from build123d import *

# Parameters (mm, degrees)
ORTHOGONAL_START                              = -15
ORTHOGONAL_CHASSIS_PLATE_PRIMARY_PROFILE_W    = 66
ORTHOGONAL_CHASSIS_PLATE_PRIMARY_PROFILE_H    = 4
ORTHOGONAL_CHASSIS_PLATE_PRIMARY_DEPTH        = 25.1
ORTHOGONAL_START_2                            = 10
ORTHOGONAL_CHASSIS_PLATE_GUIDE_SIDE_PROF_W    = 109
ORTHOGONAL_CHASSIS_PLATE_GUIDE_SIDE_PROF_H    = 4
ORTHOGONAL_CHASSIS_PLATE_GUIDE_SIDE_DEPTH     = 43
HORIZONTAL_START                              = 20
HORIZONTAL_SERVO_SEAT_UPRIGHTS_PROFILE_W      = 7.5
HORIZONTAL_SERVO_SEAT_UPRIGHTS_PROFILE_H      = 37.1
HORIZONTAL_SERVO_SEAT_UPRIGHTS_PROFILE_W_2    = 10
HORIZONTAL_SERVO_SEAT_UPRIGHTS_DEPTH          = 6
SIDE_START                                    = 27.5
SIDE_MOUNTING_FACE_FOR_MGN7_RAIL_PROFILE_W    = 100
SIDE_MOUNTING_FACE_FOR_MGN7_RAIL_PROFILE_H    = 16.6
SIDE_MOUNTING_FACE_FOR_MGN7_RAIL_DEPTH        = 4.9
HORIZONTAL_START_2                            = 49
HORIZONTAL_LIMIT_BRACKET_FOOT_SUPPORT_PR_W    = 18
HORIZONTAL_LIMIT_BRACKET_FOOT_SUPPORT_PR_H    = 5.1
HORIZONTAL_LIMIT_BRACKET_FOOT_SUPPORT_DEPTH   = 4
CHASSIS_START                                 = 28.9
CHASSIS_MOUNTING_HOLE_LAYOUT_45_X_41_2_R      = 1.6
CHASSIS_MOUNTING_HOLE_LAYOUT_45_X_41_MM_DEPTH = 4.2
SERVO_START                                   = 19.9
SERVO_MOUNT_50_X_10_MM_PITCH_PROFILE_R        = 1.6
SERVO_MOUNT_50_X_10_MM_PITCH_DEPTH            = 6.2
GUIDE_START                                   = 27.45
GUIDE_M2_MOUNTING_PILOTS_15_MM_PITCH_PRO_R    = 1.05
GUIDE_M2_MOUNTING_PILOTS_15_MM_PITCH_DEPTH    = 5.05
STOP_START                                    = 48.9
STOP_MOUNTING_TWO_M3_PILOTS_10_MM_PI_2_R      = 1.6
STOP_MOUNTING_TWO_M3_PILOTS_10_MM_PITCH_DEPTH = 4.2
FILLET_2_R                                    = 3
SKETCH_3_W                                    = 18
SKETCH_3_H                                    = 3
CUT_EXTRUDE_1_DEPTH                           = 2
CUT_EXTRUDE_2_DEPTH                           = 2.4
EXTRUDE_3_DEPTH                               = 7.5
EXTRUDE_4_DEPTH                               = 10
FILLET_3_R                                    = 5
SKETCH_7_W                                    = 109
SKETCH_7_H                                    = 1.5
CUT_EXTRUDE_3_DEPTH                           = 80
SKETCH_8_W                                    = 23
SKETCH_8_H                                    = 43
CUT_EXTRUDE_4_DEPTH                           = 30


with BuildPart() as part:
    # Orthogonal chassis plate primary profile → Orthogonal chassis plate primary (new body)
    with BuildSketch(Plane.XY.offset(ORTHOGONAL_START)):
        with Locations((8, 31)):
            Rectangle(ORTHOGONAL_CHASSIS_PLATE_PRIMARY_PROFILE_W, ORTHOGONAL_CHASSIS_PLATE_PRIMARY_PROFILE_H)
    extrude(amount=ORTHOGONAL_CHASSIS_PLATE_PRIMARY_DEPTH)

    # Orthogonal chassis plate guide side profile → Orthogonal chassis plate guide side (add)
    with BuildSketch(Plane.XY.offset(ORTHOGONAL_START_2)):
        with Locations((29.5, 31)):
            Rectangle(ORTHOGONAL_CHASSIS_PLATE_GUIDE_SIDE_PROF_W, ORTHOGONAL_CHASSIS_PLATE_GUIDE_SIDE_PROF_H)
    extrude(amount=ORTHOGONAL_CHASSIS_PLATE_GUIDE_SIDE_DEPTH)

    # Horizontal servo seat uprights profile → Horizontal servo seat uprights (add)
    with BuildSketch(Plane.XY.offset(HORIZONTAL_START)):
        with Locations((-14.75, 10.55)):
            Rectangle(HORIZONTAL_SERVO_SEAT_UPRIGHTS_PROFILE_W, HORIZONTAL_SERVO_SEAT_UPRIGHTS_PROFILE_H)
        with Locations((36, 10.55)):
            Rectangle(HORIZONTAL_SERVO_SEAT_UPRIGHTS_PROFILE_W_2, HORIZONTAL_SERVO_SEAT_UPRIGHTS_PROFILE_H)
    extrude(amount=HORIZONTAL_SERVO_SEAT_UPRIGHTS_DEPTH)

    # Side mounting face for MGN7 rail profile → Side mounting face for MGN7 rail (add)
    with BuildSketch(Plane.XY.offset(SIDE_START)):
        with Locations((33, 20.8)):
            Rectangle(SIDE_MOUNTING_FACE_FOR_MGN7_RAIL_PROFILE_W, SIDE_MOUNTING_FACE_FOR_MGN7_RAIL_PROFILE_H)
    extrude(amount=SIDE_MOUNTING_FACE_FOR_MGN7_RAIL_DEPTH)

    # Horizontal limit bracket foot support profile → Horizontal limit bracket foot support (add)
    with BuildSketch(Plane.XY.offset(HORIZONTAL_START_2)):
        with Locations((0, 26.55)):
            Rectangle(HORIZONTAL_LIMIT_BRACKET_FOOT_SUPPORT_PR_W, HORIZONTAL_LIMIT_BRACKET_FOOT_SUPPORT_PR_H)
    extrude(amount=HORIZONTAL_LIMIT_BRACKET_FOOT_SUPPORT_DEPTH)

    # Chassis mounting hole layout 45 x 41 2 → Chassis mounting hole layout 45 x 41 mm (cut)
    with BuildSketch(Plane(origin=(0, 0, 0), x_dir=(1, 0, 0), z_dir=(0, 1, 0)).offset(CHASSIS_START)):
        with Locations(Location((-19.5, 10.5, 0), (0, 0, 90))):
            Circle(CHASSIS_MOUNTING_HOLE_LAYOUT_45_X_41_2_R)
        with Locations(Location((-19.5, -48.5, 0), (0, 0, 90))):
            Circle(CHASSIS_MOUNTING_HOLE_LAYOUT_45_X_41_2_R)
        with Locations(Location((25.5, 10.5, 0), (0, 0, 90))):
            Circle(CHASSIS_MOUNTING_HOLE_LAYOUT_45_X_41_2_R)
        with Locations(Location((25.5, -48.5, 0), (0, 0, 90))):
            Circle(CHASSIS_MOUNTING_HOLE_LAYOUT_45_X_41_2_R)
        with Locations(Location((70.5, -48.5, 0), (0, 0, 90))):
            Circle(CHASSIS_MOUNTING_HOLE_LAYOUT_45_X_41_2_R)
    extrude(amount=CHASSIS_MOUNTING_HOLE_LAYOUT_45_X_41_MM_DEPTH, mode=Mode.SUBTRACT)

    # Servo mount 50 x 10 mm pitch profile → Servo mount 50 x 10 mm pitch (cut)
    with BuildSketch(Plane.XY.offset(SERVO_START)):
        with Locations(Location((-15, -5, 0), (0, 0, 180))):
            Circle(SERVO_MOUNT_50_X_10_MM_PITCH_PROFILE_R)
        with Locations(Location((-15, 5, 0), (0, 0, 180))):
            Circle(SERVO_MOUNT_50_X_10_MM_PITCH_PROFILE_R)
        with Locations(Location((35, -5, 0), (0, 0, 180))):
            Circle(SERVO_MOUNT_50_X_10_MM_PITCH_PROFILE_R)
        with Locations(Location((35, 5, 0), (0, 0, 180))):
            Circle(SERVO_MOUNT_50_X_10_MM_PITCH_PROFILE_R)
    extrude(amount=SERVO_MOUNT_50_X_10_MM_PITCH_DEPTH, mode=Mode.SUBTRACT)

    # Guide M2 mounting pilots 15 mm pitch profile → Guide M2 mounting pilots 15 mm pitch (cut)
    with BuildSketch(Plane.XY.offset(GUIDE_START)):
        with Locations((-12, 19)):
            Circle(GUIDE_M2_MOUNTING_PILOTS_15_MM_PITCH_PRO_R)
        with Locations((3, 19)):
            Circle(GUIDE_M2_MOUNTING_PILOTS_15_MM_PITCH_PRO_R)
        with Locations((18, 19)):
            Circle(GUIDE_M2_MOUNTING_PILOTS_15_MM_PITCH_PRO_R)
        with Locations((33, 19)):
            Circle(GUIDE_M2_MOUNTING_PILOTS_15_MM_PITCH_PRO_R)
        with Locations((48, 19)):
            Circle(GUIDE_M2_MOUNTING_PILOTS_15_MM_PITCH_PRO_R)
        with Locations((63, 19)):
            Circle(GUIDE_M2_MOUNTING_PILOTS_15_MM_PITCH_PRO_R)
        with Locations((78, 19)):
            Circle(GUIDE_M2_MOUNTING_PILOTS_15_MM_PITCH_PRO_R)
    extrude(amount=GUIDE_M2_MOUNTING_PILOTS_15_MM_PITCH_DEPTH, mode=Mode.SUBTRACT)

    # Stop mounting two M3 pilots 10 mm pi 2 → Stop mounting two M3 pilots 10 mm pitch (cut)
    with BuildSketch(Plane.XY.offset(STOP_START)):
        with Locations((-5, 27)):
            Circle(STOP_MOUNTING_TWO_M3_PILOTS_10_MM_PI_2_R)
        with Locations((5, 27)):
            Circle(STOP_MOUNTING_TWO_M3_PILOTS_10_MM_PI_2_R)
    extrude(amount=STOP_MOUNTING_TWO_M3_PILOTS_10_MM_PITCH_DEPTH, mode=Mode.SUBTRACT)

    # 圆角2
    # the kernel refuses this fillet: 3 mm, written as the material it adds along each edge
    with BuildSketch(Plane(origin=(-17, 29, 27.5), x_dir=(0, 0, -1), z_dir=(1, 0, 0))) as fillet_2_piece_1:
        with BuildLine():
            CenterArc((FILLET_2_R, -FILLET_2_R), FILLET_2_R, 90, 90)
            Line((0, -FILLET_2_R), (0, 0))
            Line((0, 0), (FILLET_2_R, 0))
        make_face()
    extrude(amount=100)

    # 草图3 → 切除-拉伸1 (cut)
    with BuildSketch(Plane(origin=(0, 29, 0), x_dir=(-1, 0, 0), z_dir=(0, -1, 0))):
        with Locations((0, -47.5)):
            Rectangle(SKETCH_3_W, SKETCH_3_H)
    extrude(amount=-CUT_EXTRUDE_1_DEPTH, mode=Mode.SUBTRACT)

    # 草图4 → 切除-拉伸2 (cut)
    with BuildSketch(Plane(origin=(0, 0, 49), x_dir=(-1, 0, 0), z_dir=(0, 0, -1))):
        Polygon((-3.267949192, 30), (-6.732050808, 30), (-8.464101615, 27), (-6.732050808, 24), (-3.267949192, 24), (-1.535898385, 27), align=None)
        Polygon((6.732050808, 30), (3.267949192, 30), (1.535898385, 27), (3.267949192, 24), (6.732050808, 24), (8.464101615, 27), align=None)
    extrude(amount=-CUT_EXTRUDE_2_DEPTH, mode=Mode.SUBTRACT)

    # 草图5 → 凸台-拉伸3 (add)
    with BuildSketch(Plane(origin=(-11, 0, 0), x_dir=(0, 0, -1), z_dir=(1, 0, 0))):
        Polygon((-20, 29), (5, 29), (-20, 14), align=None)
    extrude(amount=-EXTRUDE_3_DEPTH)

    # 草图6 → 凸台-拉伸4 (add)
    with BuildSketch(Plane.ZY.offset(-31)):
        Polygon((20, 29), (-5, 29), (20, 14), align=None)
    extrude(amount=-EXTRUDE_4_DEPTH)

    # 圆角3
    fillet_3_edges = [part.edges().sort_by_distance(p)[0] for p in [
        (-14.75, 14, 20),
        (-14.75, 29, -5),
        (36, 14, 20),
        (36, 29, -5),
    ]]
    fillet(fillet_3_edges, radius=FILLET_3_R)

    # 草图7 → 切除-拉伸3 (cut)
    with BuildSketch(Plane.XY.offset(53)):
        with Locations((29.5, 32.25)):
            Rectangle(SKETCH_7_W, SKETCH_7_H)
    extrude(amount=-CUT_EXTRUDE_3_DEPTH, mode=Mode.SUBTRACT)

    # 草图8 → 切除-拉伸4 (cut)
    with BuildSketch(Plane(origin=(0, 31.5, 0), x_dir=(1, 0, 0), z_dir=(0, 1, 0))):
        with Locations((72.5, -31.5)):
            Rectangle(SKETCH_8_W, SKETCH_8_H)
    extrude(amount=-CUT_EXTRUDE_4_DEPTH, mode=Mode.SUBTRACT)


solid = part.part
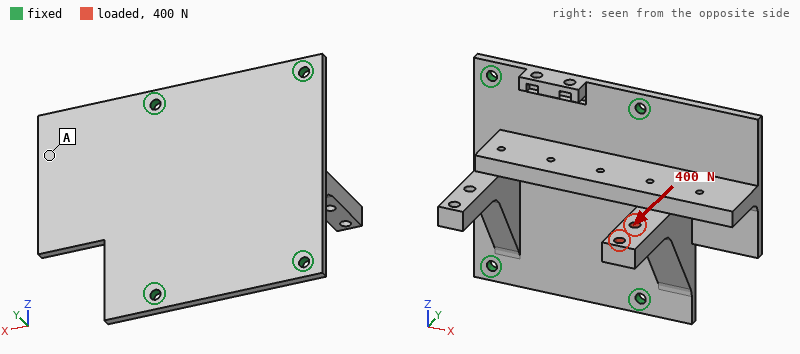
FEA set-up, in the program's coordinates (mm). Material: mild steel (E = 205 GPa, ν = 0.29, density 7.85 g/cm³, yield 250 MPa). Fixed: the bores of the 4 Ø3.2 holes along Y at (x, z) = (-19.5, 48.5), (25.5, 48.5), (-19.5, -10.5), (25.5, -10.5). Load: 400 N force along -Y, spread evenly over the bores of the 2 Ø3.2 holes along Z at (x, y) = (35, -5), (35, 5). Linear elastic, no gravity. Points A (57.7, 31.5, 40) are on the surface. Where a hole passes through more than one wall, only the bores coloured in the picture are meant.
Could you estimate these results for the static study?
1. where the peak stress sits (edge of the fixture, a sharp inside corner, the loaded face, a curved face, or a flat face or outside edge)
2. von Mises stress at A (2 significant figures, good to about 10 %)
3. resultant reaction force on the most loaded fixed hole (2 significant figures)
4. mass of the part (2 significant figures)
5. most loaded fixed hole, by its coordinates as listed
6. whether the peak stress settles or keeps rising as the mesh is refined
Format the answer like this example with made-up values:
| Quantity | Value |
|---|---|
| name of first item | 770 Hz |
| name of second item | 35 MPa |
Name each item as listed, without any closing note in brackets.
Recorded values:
| Quantity | Value |
|---|---|
| where the peak stress sits | edge of the fixture |
| von Mises stress at A | 12 MPa |
| resultant reaction force on the most loaded fixed hole | 320 N |
| mass of the part | 210 g |
| most loaded fixed hole, by its coordinates as listed | (25.5, 48.5) |
| whether the peak stress settles or keeps rising as the mesh is refined | keeps rising |
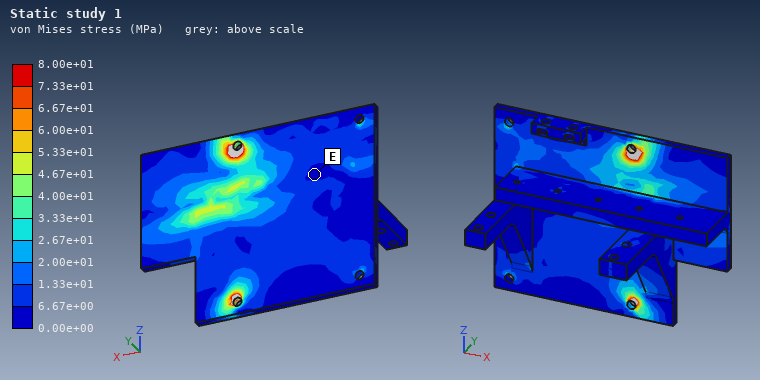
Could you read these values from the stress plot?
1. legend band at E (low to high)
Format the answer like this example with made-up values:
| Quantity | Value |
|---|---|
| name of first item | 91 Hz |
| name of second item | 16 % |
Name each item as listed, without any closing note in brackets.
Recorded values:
| Quantity | Value |
|---|---|
| legend band at E | 0.00e+00 to 6.67e+00 MPa |
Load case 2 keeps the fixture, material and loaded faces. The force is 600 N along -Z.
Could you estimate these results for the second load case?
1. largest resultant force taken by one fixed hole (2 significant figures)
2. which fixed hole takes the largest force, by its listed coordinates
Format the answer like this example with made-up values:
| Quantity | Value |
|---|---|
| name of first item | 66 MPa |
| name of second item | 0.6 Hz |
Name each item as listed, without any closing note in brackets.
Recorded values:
| Quantity | Value |
|---|---|
| largest resultant force taken by one fixed hole | 520 N |
| which fixed hole takes the largest force, by its listed coordinates | (25.5, -10.5) |
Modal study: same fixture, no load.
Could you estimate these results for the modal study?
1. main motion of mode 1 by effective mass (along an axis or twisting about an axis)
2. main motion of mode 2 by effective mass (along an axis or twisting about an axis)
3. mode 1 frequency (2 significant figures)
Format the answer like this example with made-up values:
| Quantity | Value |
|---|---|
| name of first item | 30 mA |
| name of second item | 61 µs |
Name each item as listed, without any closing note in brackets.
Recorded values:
| Quantity | Value |
|---|---|
| main motion of mode 1 by effective mass | along Y |
| main motion of mode 2 by effective mass | along Y |
| mode 1 frequency | 1700 Hz |
